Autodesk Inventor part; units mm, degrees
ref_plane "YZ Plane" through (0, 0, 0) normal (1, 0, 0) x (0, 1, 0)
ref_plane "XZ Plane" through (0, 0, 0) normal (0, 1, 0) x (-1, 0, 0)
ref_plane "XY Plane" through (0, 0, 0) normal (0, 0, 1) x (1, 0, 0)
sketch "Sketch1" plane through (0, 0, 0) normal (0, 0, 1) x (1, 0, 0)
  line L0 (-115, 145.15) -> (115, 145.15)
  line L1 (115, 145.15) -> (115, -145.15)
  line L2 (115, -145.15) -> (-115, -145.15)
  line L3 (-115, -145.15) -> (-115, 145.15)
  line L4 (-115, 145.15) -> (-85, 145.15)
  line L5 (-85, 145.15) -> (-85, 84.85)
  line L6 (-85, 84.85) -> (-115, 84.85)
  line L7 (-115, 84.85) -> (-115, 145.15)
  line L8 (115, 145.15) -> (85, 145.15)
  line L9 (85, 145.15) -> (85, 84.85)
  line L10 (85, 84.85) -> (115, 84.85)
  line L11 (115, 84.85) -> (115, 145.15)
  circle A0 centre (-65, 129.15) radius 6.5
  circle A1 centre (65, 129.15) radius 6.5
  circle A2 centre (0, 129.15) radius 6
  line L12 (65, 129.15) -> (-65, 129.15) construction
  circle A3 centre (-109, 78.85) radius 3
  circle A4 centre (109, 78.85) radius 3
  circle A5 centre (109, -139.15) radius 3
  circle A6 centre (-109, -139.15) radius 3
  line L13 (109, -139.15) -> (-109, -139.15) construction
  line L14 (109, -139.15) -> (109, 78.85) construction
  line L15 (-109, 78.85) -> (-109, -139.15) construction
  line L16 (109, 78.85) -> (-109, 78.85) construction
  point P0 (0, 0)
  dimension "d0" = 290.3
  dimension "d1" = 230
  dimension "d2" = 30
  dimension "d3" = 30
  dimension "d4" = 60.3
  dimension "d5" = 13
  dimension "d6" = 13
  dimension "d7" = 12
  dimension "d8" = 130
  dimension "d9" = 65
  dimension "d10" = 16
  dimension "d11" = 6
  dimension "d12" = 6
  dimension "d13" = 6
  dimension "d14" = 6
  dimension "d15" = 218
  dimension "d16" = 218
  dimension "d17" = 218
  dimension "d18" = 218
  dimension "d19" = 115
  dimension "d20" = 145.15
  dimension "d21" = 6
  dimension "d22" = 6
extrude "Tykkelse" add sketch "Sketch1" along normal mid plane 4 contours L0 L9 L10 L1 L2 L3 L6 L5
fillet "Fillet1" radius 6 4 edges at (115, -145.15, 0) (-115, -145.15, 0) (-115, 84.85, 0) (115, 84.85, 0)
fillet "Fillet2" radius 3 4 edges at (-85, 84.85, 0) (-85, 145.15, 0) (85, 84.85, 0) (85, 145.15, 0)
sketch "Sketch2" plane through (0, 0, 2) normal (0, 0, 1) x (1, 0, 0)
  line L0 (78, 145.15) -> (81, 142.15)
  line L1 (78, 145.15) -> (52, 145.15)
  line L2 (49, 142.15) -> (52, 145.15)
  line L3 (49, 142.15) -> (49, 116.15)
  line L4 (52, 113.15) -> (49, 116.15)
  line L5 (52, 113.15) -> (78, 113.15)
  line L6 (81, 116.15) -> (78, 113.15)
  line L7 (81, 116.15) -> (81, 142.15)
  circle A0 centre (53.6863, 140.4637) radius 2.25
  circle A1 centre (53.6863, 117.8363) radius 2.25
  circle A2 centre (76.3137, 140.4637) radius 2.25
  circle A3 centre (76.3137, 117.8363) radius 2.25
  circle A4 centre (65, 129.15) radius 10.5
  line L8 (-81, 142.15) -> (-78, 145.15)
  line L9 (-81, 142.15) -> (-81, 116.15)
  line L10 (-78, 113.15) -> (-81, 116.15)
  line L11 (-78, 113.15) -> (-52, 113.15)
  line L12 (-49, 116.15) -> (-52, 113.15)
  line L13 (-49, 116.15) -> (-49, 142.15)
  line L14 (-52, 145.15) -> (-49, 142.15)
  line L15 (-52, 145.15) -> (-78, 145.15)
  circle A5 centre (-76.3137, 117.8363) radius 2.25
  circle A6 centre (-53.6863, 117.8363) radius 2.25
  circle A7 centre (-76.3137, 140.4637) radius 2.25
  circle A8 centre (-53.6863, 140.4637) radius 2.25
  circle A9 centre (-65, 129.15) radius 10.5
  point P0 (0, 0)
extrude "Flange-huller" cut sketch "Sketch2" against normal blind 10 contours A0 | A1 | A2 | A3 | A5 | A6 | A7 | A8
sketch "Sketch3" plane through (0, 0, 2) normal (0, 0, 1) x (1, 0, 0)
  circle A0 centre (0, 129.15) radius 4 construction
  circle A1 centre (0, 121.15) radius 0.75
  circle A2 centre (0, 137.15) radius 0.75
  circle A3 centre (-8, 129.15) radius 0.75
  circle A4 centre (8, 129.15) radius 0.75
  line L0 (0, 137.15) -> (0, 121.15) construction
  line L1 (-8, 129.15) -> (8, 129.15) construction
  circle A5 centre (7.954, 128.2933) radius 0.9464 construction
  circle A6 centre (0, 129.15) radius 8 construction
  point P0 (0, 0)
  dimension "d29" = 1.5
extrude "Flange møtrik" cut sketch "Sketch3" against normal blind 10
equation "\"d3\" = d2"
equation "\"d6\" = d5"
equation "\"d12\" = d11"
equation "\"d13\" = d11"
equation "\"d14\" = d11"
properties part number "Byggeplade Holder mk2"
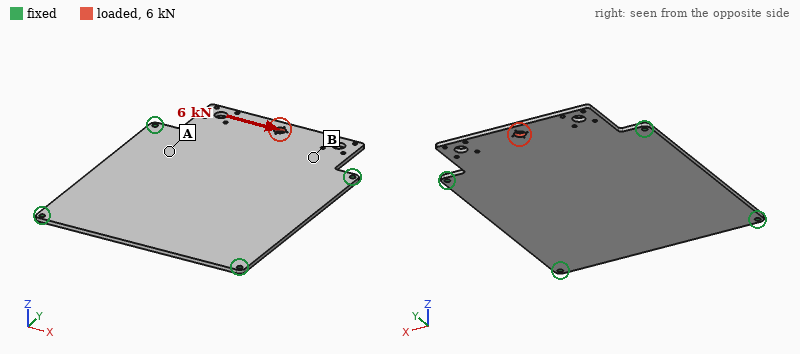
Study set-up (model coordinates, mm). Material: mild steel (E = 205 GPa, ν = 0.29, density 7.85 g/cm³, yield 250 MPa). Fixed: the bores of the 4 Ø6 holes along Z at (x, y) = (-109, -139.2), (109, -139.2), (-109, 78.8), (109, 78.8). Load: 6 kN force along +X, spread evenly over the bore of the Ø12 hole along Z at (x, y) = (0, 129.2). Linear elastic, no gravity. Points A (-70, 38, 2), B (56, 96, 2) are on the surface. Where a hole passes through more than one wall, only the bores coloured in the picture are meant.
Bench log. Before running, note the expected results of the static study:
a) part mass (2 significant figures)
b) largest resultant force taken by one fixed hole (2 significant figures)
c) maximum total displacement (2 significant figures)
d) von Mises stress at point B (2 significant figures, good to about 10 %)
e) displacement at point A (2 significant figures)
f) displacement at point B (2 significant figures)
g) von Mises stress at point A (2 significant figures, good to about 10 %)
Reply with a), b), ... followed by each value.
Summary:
a) 2.0 kg
b) 2.9 kN
c) 23 µm
d) 19 MPa
e) 6.9 µm
f) 11 µm
g) 7.3 MPa
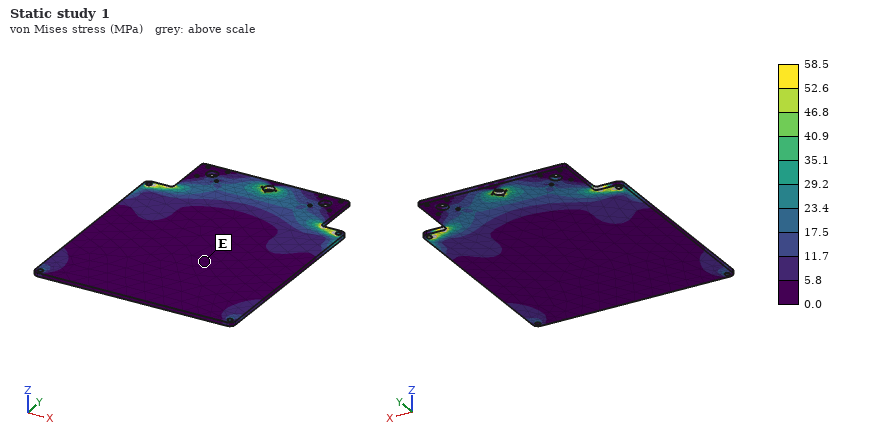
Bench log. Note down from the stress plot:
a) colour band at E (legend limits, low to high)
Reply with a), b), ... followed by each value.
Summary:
a) 0.0 to 5.8 MPa
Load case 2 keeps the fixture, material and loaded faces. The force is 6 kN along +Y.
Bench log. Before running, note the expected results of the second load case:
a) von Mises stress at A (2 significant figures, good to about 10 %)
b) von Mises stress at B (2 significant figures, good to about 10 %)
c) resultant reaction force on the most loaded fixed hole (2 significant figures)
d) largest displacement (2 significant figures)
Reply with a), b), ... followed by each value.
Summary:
a) 8.7 MPa
b) 9.3 MPa
c) 1.7 kN
d) 19 µm
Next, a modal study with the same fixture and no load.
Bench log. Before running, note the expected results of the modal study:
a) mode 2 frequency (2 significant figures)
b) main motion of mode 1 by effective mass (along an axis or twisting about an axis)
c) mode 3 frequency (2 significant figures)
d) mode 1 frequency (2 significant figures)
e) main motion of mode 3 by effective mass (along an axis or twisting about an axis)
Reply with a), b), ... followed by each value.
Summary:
a) 280 Hz
b) along Z
c) 470 Hz
d) 250 Hz
e) twisting about Y
